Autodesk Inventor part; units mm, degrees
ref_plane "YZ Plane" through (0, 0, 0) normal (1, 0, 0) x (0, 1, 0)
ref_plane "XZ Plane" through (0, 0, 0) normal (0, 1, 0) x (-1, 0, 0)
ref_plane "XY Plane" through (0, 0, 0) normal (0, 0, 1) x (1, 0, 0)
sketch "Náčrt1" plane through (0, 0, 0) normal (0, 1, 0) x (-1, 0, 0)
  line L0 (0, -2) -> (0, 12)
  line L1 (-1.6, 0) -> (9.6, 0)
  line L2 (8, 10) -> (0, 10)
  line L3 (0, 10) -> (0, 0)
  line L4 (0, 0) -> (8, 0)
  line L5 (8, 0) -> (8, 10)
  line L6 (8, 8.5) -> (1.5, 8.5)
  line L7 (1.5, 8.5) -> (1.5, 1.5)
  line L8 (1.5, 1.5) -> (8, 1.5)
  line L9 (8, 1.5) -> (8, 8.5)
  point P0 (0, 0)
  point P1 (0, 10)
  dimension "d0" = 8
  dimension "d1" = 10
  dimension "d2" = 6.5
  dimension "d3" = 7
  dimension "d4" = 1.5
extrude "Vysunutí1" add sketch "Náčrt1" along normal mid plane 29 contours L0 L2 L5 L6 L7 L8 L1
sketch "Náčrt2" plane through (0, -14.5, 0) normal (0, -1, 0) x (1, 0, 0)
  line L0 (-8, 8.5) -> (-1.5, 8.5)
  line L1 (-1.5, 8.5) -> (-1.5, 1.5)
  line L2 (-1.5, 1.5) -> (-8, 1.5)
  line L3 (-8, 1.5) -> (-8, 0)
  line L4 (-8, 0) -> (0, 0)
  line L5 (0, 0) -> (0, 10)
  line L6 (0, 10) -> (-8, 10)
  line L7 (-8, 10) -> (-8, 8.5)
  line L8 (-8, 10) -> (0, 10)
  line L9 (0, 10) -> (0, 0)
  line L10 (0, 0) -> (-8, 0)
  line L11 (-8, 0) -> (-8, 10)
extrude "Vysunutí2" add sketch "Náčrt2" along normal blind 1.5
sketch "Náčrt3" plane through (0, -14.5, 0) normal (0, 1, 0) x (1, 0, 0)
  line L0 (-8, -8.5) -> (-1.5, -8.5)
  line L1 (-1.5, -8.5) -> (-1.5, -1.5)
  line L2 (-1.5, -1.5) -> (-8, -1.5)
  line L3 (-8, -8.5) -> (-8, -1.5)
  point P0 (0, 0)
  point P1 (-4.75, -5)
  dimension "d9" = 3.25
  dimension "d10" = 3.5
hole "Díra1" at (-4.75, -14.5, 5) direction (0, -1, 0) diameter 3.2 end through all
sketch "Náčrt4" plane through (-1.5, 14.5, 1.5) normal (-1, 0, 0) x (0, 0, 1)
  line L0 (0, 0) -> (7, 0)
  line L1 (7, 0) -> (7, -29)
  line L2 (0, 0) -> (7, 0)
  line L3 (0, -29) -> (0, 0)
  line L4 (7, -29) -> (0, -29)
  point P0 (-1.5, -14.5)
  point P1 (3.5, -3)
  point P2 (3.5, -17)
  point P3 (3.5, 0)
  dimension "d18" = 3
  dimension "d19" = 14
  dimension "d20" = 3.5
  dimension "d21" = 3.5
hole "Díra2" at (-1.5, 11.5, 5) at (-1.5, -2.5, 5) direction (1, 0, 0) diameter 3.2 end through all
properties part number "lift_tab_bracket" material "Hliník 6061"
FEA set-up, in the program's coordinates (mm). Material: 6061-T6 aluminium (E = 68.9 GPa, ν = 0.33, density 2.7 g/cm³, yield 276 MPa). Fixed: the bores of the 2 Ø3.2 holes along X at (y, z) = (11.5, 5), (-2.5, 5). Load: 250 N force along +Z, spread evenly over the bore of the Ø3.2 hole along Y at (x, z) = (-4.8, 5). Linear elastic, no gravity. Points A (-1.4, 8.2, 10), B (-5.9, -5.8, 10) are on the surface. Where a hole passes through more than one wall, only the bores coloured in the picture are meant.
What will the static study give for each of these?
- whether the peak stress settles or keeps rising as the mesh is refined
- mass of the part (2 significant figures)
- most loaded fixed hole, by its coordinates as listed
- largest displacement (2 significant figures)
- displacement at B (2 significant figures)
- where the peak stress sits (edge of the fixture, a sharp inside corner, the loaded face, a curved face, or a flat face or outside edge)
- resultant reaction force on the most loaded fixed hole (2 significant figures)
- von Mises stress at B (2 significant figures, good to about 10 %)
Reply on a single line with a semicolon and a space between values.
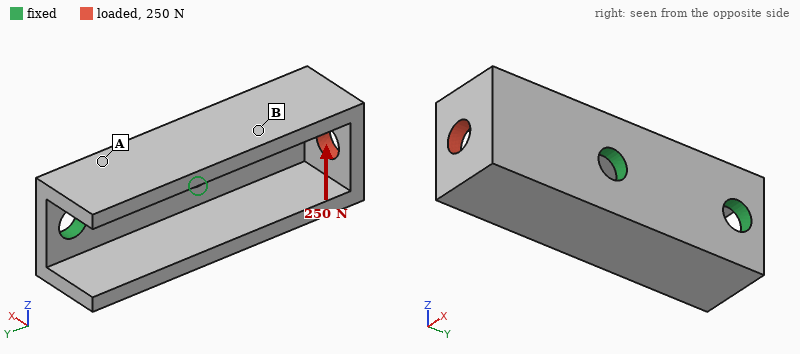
keeps rising; 2.9 g; (-2.5, 5); 0.12 mm; 0.045 mm; edge of the fixture; 370 N; 52 MPa
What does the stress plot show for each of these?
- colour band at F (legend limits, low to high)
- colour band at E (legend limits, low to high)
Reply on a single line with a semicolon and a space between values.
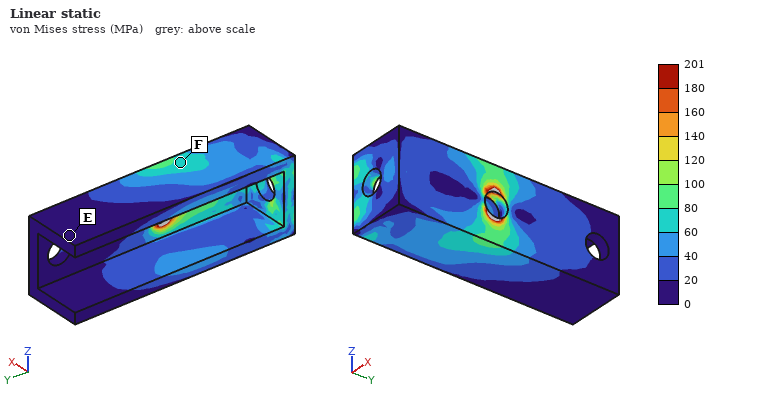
60 to 80 MPa; 0 to 20 MPa
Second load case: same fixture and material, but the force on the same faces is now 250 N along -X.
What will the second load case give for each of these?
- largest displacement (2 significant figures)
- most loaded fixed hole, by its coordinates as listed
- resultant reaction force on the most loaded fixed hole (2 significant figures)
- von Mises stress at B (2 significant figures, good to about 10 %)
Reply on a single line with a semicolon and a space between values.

56 µm; (-2.5, 5); 470 N; 44 MPa
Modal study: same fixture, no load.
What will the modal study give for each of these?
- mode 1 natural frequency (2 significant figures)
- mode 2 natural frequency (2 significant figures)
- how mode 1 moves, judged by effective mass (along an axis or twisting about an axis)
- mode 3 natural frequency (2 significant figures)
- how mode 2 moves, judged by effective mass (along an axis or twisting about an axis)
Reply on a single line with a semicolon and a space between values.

9600 Hz; 13 kHz; along Z; 15 kHz; along X
